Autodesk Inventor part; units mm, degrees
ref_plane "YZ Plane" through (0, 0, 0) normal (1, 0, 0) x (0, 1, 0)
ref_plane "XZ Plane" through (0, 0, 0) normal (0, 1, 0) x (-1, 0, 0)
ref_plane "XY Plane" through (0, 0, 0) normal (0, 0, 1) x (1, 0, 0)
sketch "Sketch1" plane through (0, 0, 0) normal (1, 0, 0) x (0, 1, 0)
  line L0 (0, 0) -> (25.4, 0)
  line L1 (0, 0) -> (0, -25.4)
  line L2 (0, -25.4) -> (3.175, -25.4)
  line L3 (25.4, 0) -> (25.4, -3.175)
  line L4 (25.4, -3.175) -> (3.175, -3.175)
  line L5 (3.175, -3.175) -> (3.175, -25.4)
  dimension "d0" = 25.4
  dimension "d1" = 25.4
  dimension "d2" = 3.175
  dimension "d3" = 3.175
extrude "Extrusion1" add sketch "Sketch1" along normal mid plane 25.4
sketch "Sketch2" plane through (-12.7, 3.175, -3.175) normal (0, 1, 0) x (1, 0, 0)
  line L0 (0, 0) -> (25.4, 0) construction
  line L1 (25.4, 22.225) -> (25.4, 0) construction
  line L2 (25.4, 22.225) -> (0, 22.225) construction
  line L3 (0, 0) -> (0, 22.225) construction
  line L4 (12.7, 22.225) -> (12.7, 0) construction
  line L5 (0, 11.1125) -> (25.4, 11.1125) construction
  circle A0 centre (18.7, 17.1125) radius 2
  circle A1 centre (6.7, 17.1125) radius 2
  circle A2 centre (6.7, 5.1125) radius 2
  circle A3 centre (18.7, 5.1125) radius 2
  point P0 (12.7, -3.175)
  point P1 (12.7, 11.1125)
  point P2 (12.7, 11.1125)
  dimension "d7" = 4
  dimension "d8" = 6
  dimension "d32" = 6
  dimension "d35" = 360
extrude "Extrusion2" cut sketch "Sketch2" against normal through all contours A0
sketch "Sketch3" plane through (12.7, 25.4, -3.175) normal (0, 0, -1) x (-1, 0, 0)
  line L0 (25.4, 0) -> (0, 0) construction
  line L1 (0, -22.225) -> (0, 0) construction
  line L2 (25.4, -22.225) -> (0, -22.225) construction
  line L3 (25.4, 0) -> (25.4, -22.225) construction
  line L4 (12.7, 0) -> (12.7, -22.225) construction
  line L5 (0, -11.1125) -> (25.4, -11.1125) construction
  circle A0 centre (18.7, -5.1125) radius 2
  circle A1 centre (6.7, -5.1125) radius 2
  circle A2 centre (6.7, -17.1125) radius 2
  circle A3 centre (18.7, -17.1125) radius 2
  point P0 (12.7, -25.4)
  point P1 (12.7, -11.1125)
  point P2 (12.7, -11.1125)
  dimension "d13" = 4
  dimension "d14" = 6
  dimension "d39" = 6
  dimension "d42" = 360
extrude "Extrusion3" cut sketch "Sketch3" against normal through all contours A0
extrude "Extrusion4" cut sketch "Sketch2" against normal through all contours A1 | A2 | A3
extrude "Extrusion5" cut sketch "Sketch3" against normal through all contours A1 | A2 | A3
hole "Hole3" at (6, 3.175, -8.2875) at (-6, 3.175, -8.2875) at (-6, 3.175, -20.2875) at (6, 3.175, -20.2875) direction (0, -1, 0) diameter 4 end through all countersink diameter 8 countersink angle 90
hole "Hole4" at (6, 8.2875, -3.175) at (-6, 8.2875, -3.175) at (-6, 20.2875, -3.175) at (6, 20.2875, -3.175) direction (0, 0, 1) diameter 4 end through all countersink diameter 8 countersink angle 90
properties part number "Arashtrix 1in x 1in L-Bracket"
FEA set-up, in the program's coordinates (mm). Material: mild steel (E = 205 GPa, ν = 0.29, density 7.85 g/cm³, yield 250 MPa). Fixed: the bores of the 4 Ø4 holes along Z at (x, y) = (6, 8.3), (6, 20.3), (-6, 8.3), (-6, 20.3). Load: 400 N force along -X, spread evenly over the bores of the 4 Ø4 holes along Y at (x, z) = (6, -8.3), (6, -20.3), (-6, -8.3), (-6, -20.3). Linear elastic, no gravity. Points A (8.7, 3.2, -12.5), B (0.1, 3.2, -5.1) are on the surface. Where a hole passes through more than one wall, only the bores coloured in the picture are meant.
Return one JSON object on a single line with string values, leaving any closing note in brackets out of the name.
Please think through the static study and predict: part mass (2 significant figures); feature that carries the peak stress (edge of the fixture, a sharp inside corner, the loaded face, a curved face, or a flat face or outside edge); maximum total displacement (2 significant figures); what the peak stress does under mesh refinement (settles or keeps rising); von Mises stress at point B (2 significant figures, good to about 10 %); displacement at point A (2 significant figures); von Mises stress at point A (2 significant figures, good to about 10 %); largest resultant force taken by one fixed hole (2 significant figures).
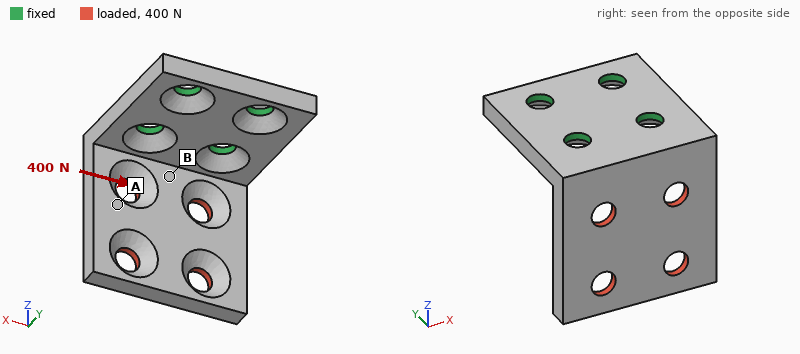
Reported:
{"part mass": "26 g", "feature that carries the peak stress": "edge of the fixture", "maximum total displacement": "21 µm", "what the peak stress does under mesh refinement": "keeps rising", "von Mises stress at point B": "38 MPa", "displacement at point A": "11 µm", "von Mises stress at point A": "13 MPa", "largest resultant force taken by one fixed hole": "530 N"}
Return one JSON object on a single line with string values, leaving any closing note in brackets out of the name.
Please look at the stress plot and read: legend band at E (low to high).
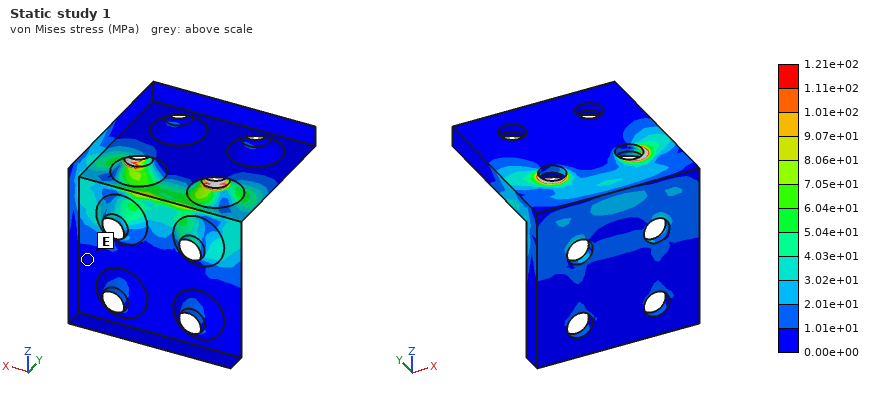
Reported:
{"legend band at E": "0.00e+00 to 1.01e+01 MPa"}
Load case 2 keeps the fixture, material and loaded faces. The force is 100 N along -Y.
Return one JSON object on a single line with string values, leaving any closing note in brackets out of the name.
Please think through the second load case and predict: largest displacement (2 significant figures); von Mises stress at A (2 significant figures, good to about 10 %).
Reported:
{"largest displacement": "37 µm", "von Mises stress at A": "9.4 MPa"}
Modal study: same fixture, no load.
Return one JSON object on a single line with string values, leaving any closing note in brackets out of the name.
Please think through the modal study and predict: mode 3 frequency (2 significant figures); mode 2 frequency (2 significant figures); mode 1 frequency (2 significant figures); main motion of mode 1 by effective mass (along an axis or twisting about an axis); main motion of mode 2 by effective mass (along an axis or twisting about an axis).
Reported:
{"mode 3 frequency": "9800 Hz", "mode 2 frequency": "6600 Hz", "mode 1 frequency": "2900 Hz", "main motion of mode 1 by effective mass": "along Y", "main motion of mode 2 by effective mass": "along X"}
